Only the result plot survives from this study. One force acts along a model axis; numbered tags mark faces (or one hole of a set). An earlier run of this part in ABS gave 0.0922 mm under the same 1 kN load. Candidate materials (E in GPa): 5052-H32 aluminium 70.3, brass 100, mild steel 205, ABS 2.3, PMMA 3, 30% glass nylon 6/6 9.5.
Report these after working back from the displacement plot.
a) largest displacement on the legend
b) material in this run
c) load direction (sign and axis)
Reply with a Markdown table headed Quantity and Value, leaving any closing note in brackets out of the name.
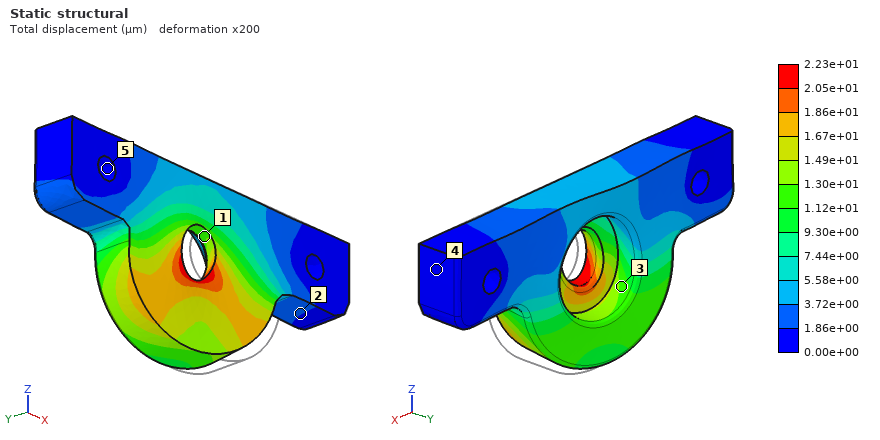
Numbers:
| Quantity | Value |
|---|---|
| largest displacement on the legend | 2.23e+01 µm |
| material in this run | 30% glass nylon 6/6 |
| load direction | -X |
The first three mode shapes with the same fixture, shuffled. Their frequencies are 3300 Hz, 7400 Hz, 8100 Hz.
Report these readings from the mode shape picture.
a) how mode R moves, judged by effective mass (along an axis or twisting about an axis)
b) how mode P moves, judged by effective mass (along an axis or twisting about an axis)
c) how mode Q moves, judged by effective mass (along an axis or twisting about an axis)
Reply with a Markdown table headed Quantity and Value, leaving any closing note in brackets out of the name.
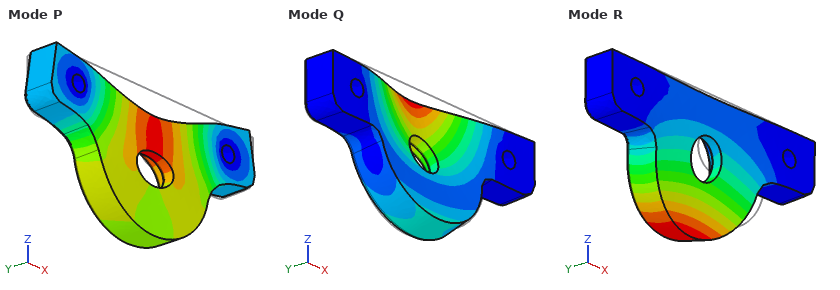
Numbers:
| Quantity | Value |
|---|---|
| how mode R moves, judged by effective mass | along Y |
| how mode P moves, judged by effective mass | along Z |
| how mode Q moves, judged by effective mass | along Y |
